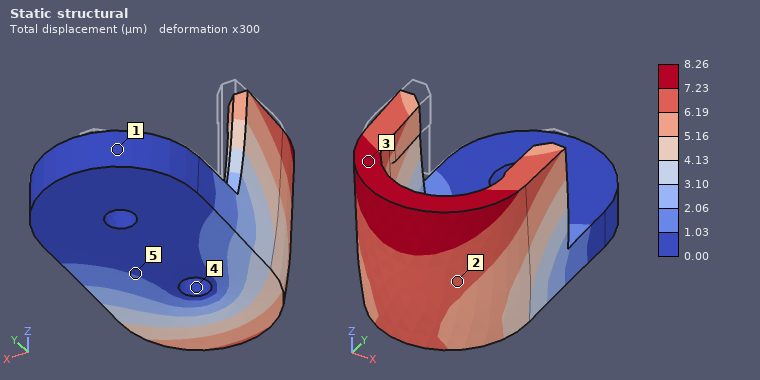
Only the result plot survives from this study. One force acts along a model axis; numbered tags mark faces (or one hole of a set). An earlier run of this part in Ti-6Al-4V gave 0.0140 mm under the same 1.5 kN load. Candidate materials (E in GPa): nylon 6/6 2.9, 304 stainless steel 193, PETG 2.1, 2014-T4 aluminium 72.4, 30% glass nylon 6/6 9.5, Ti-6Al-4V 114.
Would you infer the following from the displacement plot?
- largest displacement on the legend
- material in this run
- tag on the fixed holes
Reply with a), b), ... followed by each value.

a) 8.26 µm
b) 304 stainless steel
c) 4
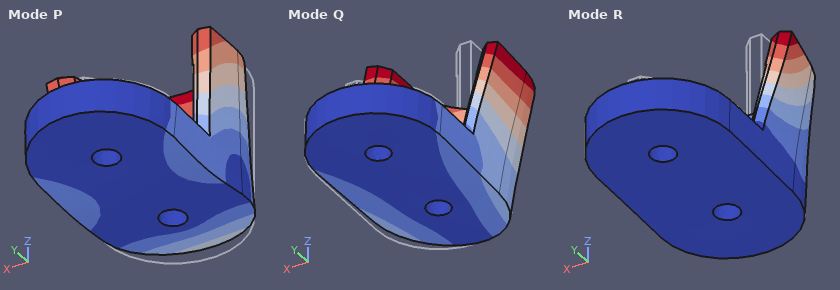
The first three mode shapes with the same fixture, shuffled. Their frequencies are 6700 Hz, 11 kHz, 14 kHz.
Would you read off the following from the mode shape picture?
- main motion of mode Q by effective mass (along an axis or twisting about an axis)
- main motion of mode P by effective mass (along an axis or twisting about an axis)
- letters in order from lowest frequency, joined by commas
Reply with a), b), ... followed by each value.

a) along X
b) along Y
c) Q, P, R
